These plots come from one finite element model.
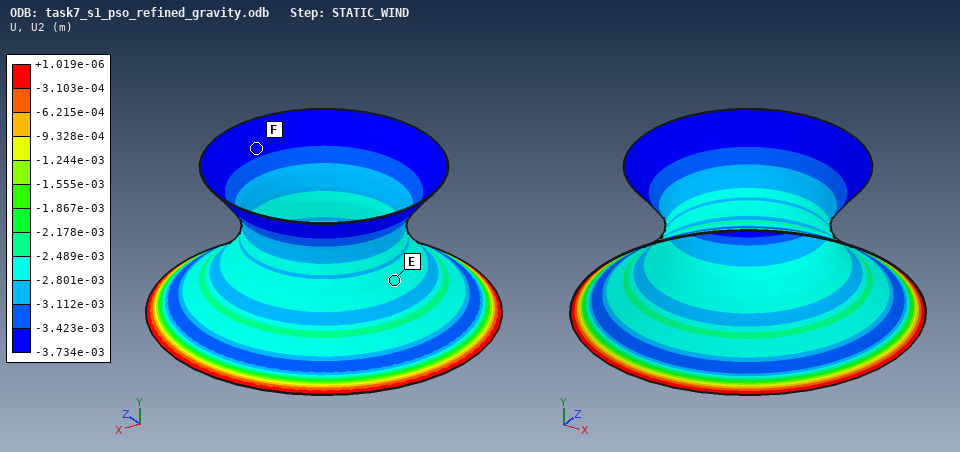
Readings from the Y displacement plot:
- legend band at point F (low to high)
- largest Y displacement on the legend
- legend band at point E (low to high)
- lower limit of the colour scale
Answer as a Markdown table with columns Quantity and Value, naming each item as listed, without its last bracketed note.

| Quantity | Value |
|---|---|
| legend band at point F | -3.734e-03 to -3.423e-03 m |
| largest Y displacement on the legend | +1.019e-06 m |
| legend band at point E | -2.801e-03 to -2.489e-03 m |
| lower limit of the colour scale | -3.734e-03 m |
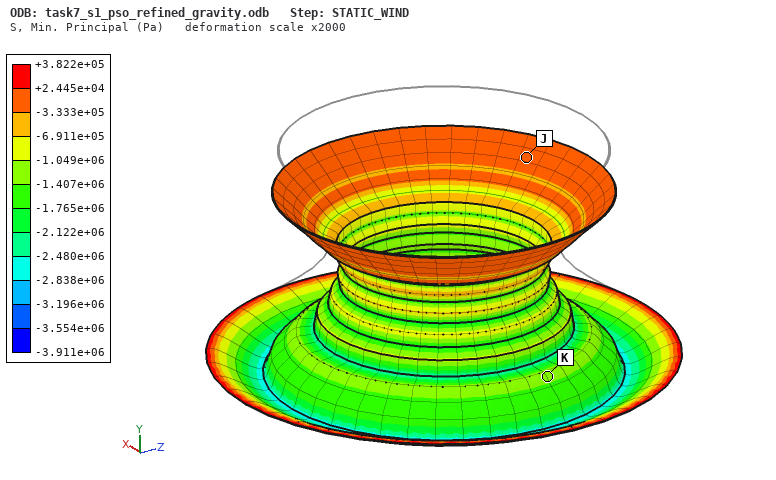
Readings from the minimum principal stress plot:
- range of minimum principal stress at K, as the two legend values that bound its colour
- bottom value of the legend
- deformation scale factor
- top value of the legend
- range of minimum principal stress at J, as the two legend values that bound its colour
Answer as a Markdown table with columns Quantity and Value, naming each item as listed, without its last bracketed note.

| Quantity | Value |
|---|---|
| range of minimum principal stress at K, as the two legend values that bound its colour | -1.407e+06 to -1.049e+06 Pa |
| bottom value of the legend | -3.911e+06 Pa |
| deformation scale factor | 2000 |
| top value of the legend | +3.822e+05 Pa |
| range of minimum principal stress at J, as the two legend values that bound its colour | -3.333e+05 to +2.445e+04 Pa |
